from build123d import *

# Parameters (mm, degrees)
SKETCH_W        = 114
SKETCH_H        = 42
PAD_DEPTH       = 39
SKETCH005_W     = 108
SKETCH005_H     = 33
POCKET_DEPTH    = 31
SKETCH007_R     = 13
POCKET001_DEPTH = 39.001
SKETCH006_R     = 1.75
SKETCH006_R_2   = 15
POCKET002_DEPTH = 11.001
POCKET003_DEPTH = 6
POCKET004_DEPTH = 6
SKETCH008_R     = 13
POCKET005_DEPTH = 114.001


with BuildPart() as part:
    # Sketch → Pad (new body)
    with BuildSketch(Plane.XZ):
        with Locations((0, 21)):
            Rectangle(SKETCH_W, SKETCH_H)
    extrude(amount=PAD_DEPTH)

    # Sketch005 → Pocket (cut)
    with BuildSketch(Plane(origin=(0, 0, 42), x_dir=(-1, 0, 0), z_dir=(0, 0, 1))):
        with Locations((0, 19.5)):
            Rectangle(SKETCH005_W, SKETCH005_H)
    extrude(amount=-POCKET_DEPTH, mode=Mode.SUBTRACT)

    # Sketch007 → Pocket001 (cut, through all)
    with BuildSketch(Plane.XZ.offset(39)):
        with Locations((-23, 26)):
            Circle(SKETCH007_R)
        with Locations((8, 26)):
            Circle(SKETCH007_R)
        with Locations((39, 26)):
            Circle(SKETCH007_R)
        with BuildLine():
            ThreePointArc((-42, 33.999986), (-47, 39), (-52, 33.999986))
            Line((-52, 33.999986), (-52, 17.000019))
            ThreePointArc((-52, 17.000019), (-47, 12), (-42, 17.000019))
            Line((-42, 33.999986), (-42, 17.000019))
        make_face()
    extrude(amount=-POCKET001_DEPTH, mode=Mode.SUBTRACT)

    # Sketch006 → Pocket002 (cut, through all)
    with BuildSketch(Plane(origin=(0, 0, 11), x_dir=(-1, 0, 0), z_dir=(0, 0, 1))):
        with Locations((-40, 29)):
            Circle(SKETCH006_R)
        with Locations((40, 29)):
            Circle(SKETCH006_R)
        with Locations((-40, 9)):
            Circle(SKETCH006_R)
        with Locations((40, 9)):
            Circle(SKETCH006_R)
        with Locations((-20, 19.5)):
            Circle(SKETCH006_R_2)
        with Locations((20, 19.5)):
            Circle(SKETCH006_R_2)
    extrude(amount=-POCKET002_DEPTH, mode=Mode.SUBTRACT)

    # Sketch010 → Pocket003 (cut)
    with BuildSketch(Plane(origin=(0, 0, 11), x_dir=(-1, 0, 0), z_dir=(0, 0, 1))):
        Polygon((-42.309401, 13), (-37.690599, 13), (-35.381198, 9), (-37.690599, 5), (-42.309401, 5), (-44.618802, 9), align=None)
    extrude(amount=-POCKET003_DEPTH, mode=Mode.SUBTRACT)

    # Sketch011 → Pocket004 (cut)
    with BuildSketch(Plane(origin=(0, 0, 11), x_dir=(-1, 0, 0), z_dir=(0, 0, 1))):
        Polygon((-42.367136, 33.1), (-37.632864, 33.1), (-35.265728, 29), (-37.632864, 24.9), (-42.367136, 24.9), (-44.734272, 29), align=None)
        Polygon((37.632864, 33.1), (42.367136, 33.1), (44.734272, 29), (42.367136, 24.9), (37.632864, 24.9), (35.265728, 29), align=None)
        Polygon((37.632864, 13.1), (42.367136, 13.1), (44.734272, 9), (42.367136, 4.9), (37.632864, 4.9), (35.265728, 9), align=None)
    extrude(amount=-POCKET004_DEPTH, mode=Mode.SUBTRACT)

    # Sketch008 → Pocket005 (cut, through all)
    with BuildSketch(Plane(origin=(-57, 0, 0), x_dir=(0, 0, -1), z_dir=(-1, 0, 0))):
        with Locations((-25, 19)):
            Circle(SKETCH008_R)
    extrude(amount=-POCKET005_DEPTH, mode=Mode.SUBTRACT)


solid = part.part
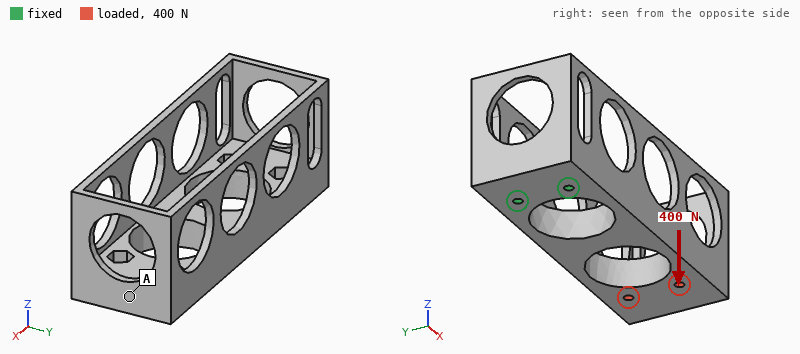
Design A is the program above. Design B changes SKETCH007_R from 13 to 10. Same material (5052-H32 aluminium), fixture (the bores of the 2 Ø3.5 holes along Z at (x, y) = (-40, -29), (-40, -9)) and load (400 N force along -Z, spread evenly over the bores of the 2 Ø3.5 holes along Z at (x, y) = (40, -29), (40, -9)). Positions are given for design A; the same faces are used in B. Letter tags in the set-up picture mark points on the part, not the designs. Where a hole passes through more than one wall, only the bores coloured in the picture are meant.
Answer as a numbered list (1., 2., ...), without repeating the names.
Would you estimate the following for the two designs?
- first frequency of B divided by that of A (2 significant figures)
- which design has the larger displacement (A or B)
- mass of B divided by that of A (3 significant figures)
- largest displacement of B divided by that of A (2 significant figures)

1. 1.0
2. A
3. 1.09
4. 0.88
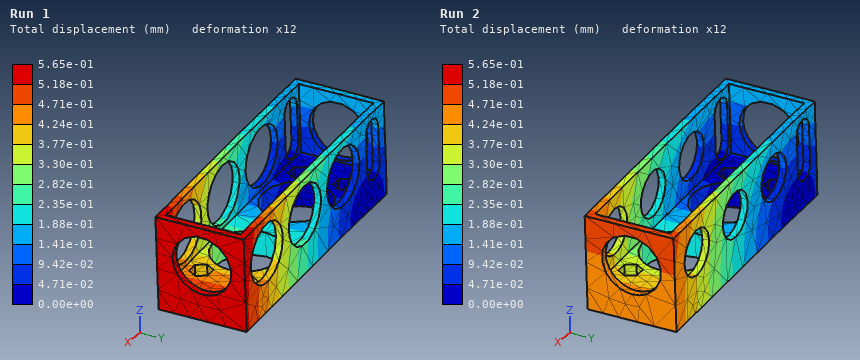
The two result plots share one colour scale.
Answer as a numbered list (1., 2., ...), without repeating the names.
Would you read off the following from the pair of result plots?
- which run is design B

1. Run 2
